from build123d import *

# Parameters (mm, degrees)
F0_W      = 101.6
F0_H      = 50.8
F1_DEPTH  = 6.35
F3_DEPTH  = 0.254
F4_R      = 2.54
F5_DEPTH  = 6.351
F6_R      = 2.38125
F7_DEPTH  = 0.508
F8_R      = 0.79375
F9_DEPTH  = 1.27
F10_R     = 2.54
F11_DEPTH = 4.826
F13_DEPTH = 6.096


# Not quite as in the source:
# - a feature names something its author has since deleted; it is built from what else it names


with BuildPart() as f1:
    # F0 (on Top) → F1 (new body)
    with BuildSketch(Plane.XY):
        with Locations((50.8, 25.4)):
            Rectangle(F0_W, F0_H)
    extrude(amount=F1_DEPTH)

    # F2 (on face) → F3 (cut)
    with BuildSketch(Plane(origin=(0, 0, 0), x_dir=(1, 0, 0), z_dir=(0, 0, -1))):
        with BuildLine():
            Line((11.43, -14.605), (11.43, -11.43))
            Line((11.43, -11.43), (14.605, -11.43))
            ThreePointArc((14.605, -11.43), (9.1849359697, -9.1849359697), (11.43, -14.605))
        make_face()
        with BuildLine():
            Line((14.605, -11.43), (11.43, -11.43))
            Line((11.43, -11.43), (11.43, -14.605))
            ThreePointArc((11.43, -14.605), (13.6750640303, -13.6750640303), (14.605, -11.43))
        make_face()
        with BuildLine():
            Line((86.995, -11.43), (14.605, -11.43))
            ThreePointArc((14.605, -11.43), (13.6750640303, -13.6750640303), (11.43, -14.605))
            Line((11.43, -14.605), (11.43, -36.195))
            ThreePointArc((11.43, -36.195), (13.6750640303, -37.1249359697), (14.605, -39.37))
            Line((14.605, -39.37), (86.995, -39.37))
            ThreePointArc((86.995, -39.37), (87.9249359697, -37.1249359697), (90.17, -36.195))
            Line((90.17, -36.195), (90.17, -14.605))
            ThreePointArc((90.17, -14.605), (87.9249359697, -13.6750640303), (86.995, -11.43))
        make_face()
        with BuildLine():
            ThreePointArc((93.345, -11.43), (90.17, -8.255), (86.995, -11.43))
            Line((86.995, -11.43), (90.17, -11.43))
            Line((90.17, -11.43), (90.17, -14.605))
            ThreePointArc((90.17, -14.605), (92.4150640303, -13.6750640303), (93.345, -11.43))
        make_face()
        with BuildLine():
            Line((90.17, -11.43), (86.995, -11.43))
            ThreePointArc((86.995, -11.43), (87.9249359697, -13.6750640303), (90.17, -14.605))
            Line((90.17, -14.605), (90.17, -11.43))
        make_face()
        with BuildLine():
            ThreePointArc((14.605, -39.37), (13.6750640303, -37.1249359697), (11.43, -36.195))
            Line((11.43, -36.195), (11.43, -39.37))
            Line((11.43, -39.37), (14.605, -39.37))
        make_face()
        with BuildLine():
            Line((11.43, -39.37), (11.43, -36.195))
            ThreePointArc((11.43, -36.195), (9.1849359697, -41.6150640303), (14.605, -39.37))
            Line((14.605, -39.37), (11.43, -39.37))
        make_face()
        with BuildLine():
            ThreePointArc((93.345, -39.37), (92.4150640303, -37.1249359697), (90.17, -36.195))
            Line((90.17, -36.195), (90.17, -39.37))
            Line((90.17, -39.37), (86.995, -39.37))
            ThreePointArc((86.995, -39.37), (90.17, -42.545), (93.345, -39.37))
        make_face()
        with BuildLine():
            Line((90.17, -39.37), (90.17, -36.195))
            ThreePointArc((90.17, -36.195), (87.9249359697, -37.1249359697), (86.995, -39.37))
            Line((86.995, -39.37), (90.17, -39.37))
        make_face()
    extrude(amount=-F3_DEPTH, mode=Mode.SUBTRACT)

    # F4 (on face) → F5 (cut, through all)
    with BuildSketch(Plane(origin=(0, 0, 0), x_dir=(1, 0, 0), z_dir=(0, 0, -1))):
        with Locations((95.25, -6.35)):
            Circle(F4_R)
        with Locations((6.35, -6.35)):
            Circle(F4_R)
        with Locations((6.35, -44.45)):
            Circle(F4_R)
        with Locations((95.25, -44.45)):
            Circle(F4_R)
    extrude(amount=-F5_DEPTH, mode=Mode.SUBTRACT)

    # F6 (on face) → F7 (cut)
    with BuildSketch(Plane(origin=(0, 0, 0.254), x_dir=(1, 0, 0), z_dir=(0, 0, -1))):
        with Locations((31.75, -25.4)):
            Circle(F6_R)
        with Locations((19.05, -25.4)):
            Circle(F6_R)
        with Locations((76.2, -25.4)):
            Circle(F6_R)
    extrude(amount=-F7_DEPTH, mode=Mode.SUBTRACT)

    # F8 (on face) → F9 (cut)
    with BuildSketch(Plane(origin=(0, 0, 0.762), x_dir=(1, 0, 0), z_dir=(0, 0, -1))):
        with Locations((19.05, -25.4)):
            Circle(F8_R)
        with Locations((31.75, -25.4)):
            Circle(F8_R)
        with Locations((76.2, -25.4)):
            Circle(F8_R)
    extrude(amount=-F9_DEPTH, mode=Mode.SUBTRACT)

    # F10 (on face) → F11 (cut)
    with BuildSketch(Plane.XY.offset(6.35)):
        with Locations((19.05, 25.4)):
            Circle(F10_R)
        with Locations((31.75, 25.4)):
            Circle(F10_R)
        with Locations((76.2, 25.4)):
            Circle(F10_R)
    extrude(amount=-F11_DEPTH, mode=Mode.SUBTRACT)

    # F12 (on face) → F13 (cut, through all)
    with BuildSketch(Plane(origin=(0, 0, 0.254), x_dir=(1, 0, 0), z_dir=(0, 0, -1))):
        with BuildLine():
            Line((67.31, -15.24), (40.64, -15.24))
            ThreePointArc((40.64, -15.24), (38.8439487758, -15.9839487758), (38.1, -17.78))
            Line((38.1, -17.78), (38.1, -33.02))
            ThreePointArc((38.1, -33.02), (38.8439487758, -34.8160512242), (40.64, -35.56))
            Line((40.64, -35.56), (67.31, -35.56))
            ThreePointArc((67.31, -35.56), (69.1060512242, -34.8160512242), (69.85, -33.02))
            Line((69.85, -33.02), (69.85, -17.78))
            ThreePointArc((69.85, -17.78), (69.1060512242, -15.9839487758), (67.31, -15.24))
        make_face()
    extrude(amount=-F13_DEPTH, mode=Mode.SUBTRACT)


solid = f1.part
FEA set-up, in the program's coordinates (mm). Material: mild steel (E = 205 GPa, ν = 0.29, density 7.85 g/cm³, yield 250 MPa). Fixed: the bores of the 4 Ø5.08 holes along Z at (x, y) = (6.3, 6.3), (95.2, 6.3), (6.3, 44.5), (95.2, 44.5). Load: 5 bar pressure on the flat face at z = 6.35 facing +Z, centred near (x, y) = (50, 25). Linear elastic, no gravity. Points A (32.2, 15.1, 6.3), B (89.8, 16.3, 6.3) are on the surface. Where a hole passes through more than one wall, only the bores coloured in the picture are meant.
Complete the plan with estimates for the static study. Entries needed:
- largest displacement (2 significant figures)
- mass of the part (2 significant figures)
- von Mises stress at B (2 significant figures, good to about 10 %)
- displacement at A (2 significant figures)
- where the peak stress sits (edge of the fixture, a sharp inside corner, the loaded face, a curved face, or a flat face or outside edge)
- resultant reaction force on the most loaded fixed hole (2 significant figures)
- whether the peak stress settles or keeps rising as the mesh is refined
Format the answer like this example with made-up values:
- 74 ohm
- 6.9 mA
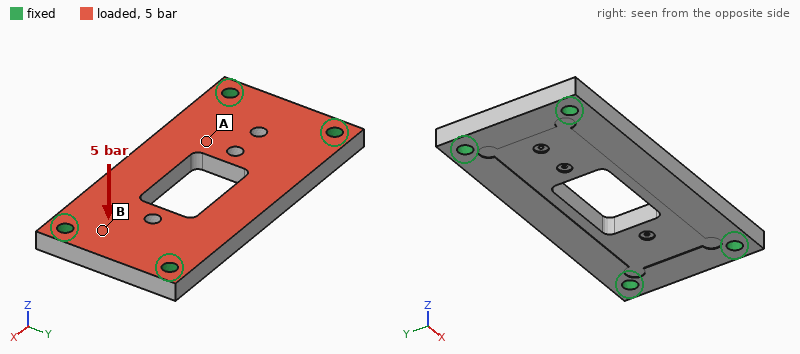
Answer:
- 21 µm
- 220 g
- 18 MPa
- 15 µm
- edge of the fixture
- 550 N
- keeps rising
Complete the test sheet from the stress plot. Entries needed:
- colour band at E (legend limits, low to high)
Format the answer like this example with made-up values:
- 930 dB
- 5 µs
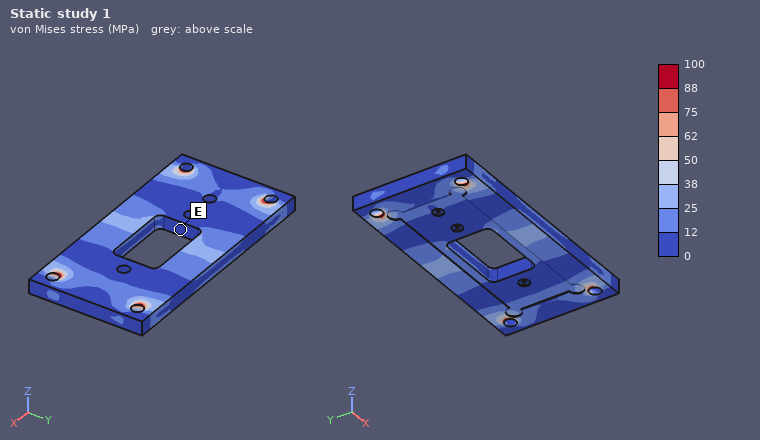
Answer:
- 0 to 12 MPa
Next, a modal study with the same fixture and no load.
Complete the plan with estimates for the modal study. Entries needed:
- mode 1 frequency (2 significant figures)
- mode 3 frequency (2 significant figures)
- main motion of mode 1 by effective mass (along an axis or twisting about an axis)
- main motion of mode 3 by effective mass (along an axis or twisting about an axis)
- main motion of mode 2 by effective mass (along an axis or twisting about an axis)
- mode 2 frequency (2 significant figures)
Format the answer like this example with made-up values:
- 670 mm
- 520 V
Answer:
- 4100 Hz
- 9600 Hz
- along Z
- twisting about Y
- twisting about X
- 5700 Hz
